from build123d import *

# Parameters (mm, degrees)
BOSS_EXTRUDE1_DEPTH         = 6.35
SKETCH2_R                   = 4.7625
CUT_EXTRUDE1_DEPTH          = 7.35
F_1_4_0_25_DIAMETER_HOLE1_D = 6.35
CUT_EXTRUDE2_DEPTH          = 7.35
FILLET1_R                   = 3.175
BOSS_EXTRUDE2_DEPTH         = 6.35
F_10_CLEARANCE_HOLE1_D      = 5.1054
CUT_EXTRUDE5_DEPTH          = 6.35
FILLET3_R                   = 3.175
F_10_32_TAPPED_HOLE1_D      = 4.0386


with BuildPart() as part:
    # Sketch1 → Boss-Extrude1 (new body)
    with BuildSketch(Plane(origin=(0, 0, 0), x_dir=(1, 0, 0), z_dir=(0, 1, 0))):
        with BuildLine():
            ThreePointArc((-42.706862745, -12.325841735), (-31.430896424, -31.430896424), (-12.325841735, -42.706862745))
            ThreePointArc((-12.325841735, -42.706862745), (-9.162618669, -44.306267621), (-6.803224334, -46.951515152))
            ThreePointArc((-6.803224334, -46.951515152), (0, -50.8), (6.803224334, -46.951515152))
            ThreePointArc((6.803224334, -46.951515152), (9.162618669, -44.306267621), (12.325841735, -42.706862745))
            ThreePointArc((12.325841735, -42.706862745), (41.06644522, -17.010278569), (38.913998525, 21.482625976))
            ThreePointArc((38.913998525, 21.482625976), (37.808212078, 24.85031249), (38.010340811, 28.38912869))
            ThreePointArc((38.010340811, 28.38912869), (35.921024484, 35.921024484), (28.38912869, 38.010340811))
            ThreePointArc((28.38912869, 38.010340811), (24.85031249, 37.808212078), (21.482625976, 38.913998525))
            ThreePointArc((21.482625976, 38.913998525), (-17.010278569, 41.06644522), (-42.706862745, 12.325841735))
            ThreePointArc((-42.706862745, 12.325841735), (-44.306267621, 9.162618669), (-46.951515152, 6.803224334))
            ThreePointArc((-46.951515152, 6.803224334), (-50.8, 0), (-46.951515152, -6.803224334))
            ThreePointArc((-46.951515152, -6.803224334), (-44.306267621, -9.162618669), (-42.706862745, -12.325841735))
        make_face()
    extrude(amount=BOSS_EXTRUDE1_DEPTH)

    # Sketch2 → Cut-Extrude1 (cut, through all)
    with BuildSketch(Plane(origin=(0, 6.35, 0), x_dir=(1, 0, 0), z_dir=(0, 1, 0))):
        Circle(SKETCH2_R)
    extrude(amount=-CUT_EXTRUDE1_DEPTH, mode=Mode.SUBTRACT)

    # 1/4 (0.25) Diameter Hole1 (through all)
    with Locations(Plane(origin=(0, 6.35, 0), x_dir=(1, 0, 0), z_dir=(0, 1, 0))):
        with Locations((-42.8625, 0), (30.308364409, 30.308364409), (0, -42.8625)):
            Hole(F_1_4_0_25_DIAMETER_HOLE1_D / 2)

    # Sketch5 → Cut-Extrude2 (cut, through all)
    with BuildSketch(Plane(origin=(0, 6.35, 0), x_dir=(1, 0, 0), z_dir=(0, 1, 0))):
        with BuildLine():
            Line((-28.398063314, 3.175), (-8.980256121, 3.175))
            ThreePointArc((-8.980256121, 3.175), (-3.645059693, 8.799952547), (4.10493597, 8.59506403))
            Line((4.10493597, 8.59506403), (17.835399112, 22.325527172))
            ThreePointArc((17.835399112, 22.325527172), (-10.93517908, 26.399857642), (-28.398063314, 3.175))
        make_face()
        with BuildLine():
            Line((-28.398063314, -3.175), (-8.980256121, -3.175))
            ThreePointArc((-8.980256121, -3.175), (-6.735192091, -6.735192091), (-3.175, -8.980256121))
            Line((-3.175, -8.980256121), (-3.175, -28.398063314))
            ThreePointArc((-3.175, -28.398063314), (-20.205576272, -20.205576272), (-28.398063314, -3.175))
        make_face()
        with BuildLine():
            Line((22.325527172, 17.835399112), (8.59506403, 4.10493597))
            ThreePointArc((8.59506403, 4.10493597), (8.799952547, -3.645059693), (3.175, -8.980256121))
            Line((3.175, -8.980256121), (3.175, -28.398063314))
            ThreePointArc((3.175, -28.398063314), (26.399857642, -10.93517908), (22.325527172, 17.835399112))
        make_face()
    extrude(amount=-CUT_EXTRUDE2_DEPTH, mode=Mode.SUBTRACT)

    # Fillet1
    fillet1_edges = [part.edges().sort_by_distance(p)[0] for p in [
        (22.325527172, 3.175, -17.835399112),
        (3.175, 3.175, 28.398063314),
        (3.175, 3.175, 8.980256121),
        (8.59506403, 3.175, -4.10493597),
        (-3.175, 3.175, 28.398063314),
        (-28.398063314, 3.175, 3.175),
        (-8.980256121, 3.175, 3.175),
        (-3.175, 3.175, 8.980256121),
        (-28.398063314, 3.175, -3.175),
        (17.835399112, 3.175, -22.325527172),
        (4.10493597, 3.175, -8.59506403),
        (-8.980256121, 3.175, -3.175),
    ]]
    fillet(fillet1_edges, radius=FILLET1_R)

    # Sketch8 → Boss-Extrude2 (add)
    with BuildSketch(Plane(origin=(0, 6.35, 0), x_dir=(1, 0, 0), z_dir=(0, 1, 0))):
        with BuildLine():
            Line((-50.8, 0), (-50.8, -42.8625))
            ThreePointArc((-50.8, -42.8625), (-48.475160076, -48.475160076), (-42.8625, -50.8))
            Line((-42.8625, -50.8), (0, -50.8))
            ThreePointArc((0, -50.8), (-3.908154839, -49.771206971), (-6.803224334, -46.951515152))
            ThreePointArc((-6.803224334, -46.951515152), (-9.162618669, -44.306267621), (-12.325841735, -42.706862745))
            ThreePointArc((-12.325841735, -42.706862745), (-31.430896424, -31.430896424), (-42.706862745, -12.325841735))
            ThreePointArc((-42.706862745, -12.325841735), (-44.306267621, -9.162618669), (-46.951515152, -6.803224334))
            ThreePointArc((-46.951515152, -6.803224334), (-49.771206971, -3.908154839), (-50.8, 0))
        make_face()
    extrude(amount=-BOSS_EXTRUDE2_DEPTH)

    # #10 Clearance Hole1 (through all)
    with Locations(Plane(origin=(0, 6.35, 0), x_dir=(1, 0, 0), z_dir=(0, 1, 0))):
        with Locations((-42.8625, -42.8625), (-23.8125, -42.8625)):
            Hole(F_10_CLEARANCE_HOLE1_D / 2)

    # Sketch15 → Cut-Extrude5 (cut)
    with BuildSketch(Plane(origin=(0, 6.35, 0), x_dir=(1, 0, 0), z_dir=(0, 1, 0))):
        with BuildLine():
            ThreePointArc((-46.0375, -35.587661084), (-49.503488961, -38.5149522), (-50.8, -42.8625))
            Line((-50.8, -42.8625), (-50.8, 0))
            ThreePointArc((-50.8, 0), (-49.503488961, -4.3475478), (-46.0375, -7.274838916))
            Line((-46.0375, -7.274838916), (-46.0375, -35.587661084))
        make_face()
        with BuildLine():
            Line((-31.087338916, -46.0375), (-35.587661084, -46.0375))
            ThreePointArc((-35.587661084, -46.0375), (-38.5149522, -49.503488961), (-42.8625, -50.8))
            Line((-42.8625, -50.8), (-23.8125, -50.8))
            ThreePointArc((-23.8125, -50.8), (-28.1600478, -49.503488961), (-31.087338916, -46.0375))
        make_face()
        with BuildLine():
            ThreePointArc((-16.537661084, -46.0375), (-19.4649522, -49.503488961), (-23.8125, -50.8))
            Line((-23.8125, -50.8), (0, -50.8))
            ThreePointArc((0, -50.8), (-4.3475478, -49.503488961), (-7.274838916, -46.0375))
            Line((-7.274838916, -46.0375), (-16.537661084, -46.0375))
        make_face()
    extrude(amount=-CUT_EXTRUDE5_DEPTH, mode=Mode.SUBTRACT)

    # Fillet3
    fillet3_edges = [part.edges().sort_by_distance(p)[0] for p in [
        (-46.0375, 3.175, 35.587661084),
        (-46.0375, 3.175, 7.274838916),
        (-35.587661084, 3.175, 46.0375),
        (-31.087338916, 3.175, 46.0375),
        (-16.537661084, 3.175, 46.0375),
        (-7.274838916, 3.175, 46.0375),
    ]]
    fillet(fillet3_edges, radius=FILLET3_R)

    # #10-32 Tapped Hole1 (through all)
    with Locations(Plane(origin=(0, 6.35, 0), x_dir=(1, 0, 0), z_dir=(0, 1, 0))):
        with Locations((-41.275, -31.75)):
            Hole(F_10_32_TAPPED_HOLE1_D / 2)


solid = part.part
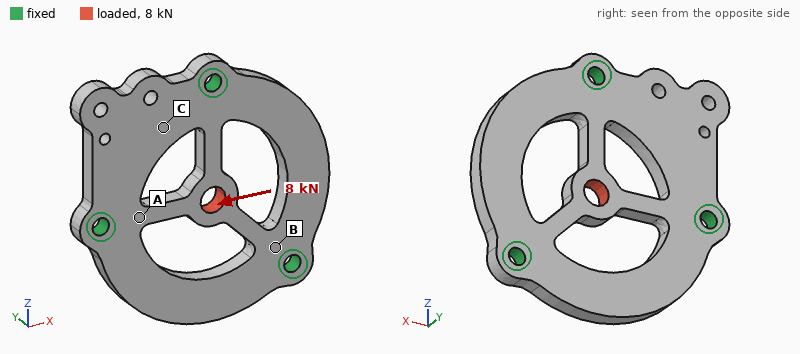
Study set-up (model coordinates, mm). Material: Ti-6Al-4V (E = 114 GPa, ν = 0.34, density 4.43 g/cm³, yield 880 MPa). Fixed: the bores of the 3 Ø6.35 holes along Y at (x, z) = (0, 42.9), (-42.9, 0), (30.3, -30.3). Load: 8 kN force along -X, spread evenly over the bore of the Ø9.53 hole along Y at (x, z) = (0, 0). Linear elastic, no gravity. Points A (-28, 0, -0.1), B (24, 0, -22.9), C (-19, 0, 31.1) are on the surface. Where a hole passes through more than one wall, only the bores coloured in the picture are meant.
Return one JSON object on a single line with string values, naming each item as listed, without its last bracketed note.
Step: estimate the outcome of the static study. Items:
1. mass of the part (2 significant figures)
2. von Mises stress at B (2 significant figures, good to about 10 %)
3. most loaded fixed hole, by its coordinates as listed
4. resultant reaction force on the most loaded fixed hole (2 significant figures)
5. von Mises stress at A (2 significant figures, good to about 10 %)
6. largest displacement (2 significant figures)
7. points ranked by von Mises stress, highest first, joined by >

{"mass of the part": "140 g", "von Mises stress at B": "48 MPa", "most loaded fixed hole, by its coordinates as listed": "(-42.9, 0)", "resultant reaction force on the most loaded fixed hole": "5.1 kN", "von Mises stress at A": "97 MPa", "largest displacement": "66 µm", "points ranked by von Mises stress, highest first, joined by >": "A > B > C"}
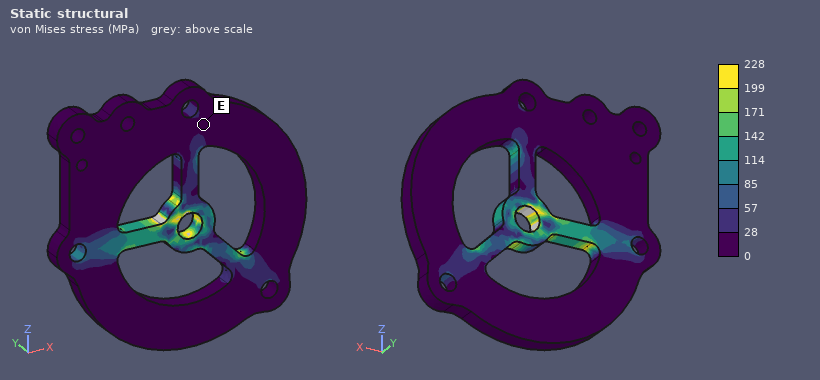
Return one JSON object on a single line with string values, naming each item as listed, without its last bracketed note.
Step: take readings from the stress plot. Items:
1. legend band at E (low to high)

{"legend band at E": "0 to 28 MPa"}
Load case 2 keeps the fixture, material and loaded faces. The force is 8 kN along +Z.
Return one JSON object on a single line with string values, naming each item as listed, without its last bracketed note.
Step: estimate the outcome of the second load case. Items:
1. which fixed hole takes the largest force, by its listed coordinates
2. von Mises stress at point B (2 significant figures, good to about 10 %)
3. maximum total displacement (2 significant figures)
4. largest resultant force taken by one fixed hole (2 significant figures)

{"which fixed hole takes the largest force, by its listed coordinates": "(0, 42.9)", "von Mises stress at point B": "38 MPa", "maximum total displacement": "66 µm", "largest resultant force taken by one fixed hole": "5.1 kN"}
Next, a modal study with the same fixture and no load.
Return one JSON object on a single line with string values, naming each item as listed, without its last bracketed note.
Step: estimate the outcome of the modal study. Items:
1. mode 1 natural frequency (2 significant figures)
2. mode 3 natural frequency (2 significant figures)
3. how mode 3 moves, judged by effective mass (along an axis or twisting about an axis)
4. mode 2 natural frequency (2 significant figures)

{"mode 1 natural frequency": "3600 Hz", "mode 3 natural frequency": "4000 Hz", "how mode 3 moves, judged by effective mass": "along Y", "mode 2 natural frequency": "3800 Hz"}
